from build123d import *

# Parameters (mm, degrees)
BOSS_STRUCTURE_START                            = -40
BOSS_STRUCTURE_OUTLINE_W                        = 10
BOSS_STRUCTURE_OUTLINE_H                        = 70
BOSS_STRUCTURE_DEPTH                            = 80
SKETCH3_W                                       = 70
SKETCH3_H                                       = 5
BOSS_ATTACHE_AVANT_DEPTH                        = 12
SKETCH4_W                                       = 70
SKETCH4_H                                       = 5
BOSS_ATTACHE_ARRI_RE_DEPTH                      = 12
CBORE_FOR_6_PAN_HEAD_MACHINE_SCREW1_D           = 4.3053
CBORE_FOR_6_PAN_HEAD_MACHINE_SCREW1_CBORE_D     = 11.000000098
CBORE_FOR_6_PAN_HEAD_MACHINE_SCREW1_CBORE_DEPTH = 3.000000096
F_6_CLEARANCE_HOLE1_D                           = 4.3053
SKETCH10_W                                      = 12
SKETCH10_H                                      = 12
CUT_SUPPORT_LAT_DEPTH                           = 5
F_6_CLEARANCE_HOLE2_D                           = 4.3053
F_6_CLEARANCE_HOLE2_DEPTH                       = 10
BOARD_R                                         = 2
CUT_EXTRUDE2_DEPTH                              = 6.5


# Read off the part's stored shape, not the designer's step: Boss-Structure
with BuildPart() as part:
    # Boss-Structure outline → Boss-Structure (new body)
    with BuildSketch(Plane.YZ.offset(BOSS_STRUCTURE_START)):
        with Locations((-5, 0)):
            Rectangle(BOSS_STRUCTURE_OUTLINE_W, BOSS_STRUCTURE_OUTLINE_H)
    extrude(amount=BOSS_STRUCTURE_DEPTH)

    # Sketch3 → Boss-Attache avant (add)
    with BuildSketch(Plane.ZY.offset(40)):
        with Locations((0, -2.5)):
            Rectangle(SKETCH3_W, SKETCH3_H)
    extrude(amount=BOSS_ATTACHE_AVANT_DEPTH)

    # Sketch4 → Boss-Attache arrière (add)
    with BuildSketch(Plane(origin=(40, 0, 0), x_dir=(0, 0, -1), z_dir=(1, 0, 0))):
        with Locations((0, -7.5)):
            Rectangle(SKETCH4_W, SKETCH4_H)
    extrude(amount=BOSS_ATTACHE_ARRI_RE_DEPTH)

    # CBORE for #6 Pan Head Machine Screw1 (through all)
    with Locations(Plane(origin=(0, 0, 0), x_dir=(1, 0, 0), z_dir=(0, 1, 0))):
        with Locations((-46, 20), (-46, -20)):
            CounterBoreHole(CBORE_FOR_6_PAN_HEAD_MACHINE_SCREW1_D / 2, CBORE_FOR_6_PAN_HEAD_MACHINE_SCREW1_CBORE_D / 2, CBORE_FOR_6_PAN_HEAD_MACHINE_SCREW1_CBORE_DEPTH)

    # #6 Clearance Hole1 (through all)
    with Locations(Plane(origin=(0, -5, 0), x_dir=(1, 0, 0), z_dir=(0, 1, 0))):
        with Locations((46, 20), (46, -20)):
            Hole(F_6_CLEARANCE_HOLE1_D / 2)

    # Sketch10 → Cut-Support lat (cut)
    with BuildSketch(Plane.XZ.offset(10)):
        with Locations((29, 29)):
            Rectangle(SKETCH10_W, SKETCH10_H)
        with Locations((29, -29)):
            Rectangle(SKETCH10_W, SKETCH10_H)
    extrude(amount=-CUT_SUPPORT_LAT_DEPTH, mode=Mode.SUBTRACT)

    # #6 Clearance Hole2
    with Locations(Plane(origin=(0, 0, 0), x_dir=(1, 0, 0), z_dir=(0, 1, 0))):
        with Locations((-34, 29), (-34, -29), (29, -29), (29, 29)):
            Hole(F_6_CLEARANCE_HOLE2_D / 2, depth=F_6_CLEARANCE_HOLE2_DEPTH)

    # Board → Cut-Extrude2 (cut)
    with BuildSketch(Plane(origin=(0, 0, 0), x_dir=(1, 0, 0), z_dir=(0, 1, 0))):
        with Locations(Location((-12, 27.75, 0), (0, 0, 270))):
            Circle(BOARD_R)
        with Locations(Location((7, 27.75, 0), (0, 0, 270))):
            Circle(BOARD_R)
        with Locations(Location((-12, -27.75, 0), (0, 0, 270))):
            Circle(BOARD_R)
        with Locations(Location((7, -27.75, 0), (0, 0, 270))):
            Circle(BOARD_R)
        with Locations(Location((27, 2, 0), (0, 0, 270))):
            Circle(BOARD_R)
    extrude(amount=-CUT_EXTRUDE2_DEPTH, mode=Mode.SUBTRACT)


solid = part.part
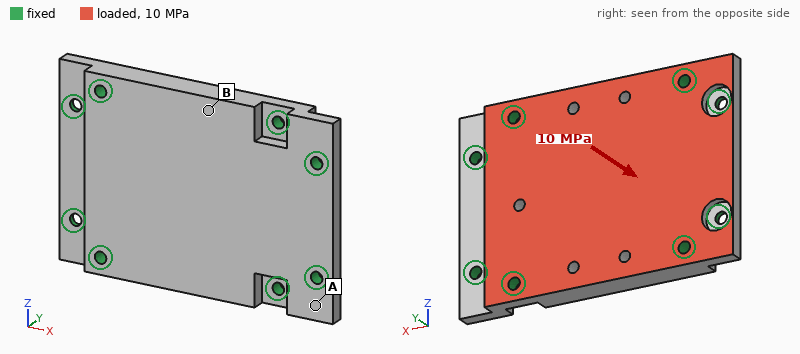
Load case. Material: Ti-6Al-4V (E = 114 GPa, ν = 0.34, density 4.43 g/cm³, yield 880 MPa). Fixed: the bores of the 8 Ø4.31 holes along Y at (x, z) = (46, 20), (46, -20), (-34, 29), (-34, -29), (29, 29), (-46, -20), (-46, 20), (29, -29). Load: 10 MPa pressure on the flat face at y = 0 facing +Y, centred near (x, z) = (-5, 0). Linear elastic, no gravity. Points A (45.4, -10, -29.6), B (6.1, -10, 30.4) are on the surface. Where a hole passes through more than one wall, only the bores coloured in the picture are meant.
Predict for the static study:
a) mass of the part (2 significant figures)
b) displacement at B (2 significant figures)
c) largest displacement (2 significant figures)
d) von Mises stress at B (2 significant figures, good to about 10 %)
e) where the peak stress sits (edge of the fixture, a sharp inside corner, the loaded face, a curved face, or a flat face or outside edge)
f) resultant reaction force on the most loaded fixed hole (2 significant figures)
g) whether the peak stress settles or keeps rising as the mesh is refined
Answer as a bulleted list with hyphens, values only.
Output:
- 270 g
- 0.099 mm
- 0.15 mm
- 170 MPa
- edge of the fixture
- 15 kN
- keeps rising
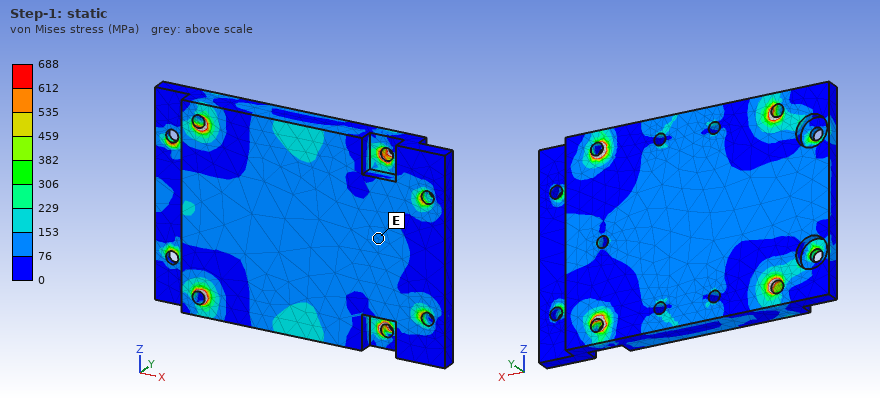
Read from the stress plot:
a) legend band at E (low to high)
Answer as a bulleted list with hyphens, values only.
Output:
- 76 to 153 MPa
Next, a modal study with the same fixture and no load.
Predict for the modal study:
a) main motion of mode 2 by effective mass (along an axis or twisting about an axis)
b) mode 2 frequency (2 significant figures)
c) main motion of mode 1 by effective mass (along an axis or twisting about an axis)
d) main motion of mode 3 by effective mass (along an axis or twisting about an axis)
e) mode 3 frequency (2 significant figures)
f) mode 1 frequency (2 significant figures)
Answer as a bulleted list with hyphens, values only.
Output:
- twisting about X
- 11 kHz
- along Y
- twisting about Z
- 13 kHz
- 7300 Hz
